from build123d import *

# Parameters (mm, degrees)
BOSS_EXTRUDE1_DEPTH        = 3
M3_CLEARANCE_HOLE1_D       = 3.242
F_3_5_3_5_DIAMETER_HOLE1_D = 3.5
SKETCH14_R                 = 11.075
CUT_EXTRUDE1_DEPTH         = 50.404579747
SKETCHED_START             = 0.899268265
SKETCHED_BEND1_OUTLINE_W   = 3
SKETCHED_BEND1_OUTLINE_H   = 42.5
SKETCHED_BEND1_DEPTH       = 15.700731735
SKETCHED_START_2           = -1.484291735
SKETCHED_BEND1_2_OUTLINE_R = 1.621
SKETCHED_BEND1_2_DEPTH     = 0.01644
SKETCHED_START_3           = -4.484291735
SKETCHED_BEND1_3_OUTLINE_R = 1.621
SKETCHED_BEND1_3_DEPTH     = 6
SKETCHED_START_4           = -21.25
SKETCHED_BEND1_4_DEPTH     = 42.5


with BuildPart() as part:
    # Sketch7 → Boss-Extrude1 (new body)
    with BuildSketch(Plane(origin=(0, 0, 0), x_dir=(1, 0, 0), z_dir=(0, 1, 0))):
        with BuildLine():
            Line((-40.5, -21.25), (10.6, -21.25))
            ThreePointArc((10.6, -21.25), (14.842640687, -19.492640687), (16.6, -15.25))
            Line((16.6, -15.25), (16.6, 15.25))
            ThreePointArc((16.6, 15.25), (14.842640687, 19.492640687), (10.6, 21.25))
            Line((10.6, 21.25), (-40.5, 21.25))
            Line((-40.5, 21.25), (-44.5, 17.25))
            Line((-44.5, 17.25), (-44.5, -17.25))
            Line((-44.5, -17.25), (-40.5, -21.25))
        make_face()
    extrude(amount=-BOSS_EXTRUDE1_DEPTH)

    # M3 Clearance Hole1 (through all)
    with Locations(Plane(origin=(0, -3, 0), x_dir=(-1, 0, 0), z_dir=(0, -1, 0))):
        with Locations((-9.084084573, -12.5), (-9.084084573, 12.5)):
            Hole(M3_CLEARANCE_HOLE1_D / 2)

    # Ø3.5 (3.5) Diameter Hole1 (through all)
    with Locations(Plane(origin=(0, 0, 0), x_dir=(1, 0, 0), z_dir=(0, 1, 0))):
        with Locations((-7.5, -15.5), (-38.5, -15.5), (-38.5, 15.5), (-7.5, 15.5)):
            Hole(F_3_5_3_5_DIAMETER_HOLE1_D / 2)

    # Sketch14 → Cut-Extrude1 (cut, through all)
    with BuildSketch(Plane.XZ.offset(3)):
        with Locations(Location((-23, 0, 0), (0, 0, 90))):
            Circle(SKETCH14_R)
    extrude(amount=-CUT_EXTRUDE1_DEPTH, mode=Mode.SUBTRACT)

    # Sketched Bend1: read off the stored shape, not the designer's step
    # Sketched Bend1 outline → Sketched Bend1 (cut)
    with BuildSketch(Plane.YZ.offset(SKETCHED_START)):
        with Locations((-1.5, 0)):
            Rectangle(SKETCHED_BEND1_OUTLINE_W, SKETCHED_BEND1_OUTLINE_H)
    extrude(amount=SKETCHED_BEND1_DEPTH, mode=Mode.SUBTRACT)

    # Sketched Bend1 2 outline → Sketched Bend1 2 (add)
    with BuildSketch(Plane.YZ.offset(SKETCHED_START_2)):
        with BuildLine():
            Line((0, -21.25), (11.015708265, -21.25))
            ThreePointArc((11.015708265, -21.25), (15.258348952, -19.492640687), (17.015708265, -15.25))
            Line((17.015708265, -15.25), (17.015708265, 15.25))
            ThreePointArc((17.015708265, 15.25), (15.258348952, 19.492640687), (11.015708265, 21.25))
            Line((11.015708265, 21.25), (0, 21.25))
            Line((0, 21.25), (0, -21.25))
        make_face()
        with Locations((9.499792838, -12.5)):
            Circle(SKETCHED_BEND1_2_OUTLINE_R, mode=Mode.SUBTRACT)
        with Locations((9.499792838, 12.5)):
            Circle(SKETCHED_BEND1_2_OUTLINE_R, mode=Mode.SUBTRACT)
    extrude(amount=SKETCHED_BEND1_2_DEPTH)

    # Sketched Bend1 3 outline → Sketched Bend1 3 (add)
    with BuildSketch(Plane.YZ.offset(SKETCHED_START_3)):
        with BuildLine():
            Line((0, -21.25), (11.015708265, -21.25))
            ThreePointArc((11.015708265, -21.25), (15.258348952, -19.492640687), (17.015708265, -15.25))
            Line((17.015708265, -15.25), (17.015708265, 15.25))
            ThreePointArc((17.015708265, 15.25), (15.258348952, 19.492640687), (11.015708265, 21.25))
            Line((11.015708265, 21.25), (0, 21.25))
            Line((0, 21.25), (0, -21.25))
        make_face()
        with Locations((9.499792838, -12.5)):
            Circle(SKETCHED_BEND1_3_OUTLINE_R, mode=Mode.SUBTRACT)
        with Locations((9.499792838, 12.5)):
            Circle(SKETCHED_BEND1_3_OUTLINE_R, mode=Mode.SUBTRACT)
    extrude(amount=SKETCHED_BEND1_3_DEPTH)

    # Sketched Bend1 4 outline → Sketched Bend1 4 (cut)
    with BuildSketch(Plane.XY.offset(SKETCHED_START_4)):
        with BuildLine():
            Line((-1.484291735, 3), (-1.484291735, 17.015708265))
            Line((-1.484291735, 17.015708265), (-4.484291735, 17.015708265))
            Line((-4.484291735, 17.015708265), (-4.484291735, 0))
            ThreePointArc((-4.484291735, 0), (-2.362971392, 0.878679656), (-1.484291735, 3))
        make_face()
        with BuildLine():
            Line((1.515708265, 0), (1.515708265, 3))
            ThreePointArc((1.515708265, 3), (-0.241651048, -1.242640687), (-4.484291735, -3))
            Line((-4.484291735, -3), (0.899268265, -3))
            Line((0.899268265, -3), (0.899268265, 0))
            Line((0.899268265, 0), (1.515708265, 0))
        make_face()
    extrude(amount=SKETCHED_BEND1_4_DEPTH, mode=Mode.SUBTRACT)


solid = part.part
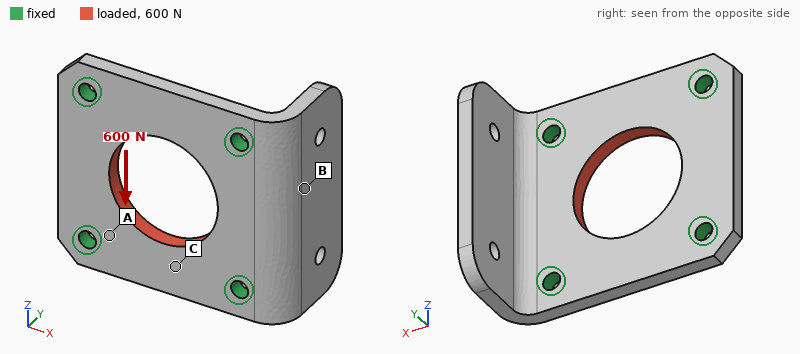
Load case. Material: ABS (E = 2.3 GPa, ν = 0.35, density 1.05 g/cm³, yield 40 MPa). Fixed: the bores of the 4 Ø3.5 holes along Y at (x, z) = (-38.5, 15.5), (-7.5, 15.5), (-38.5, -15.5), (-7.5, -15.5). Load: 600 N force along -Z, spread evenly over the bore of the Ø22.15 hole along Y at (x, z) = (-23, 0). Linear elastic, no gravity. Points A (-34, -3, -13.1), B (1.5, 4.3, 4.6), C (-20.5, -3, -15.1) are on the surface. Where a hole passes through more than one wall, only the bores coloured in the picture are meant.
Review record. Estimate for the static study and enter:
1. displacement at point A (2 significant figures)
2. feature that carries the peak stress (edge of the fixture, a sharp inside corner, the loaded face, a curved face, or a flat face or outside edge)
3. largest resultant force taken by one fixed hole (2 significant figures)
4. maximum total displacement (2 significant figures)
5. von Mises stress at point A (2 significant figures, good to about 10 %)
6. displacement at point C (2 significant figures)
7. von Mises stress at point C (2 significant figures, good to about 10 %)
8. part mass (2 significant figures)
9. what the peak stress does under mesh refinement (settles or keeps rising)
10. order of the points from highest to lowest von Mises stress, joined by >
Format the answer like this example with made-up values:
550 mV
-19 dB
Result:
18 µm
edge of the fixture
160 N
53 µm
4.6 MPa
47 µm
2.5 MPa
6.7 g
keeps rising
A > C > B
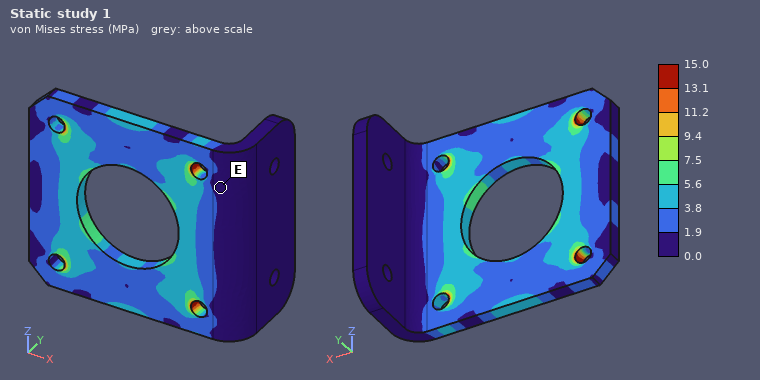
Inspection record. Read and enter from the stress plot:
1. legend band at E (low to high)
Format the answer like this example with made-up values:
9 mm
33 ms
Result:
0.0 to 1.9 MPa
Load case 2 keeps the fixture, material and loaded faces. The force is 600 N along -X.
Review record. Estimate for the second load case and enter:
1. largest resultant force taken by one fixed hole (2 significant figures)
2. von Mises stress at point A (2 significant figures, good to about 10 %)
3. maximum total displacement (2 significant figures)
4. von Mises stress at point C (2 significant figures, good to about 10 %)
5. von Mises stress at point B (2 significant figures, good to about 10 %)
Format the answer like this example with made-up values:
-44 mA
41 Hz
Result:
150 N
4.8 MPa
55 µm
3.4 MPa
1.6 MPa
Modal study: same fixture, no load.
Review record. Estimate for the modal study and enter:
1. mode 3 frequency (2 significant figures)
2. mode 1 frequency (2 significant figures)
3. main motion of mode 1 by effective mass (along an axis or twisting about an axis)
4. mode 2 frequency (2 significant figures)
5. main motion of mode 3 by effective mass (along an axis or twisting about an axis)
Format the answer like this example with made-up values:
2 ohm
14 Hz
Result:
4400 Hz
1400 Hz
along X
2400 Hz
along Y
